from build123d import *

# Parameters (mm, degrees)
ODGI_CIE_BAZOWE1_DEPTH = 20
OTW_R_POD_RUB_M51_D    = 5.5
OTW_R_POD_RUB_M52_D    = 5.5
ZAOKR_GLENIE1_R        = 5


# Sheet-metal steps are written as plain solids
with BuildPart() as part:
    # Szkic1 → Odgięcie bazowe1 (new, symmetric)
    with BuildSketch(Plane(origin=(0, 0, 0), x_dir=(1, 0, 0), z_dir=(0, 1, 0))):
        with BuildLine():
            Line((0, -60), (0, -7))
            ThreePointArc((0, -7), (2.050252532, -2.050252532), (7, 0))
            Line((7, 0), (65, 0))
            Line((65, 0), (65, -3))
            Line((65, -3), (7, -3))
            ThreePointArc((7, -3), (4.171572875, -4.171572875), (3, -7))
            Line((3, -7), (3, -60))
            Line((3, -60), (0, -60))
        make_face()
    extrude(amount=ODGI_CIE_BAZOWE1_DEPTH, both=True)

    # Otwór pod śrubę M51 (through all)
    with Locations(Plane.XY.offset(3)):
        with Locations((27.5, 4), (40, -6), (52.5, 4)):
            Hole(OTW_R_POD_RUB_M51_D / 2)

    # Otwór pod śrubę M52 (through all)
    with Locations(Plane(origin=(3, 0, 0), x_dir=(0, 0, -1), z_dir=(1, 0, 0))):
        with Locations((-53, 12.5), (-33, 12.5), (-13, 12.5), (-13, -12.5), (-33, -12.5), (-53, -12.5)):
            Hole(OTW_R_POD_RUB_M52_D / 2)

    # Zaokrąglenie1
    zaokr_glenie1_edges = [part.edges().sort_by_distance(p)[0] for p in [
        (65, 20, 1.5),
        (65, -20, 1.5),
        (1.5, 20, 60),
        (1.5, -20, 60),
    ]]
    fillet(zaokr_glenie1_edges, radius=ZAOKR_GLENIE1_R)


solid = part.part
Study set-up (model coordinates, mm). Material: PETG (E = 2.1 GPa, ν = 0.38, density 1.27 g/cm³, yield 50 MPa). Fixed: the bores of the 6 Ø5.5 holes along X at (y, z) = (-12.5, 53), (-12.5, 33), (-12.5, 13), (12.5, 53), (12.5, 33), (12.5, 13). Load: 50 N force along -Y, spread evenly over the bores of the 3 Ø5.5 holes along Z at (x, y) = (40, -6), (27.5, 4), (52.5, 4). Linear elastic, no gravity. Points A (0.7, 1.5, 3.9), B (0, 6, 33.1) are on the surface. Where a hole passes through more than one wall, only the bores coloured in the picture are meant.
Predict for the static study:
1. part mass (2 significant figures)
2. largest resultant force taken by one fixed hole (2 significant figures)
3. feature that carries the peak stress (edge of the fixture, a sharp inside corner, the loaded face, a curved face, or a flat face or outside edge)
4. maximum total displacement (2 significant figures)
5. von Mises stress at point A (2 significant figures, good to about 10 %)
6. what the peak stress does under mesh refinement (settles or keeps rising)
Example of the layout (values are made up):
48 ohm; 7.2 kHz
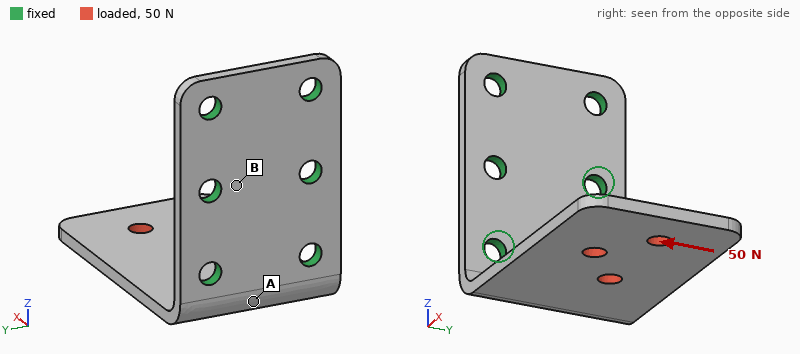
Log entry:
17 g; 78 N; edge of the fixture; 0.98 mm; 4.6 MPa; keeps rising
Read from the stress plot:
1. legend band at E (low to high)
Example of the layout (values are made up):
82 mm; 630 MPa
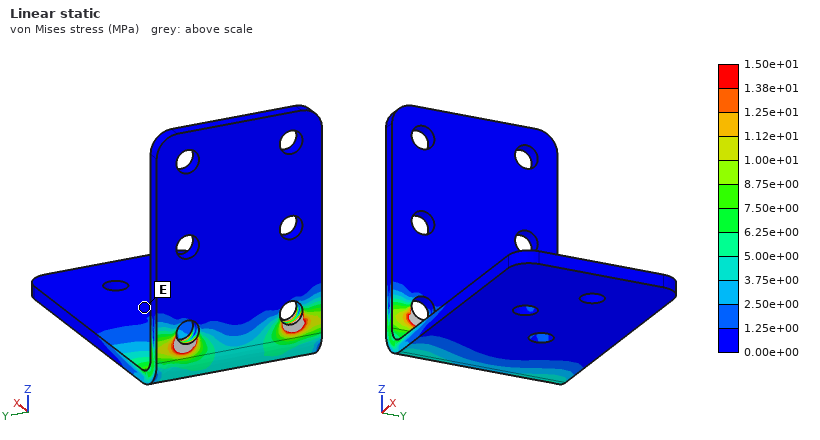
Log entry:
0.00e+00 to 1.25e+00 MPa
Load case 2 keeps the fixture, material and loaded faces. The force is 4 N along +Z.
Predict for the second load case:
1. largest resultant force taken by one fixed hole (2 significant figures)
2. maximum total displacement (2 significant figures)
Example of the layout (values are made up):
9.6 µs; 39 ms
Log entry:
2.1 N; 1.2 mm
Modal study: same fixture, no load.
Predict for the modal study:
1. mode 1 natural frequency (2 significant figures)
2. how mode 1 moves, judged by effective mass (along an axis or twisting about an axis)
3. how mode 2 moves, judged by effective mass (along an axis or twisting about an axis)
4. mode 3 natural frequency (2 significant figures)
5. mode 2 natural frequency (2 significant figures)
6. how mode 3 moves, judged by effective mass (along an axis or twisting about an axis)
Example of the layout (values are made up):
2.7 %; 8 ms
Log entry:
130 Hz; along Z; along Y; 610 Hz; 440 Hz; along Y
